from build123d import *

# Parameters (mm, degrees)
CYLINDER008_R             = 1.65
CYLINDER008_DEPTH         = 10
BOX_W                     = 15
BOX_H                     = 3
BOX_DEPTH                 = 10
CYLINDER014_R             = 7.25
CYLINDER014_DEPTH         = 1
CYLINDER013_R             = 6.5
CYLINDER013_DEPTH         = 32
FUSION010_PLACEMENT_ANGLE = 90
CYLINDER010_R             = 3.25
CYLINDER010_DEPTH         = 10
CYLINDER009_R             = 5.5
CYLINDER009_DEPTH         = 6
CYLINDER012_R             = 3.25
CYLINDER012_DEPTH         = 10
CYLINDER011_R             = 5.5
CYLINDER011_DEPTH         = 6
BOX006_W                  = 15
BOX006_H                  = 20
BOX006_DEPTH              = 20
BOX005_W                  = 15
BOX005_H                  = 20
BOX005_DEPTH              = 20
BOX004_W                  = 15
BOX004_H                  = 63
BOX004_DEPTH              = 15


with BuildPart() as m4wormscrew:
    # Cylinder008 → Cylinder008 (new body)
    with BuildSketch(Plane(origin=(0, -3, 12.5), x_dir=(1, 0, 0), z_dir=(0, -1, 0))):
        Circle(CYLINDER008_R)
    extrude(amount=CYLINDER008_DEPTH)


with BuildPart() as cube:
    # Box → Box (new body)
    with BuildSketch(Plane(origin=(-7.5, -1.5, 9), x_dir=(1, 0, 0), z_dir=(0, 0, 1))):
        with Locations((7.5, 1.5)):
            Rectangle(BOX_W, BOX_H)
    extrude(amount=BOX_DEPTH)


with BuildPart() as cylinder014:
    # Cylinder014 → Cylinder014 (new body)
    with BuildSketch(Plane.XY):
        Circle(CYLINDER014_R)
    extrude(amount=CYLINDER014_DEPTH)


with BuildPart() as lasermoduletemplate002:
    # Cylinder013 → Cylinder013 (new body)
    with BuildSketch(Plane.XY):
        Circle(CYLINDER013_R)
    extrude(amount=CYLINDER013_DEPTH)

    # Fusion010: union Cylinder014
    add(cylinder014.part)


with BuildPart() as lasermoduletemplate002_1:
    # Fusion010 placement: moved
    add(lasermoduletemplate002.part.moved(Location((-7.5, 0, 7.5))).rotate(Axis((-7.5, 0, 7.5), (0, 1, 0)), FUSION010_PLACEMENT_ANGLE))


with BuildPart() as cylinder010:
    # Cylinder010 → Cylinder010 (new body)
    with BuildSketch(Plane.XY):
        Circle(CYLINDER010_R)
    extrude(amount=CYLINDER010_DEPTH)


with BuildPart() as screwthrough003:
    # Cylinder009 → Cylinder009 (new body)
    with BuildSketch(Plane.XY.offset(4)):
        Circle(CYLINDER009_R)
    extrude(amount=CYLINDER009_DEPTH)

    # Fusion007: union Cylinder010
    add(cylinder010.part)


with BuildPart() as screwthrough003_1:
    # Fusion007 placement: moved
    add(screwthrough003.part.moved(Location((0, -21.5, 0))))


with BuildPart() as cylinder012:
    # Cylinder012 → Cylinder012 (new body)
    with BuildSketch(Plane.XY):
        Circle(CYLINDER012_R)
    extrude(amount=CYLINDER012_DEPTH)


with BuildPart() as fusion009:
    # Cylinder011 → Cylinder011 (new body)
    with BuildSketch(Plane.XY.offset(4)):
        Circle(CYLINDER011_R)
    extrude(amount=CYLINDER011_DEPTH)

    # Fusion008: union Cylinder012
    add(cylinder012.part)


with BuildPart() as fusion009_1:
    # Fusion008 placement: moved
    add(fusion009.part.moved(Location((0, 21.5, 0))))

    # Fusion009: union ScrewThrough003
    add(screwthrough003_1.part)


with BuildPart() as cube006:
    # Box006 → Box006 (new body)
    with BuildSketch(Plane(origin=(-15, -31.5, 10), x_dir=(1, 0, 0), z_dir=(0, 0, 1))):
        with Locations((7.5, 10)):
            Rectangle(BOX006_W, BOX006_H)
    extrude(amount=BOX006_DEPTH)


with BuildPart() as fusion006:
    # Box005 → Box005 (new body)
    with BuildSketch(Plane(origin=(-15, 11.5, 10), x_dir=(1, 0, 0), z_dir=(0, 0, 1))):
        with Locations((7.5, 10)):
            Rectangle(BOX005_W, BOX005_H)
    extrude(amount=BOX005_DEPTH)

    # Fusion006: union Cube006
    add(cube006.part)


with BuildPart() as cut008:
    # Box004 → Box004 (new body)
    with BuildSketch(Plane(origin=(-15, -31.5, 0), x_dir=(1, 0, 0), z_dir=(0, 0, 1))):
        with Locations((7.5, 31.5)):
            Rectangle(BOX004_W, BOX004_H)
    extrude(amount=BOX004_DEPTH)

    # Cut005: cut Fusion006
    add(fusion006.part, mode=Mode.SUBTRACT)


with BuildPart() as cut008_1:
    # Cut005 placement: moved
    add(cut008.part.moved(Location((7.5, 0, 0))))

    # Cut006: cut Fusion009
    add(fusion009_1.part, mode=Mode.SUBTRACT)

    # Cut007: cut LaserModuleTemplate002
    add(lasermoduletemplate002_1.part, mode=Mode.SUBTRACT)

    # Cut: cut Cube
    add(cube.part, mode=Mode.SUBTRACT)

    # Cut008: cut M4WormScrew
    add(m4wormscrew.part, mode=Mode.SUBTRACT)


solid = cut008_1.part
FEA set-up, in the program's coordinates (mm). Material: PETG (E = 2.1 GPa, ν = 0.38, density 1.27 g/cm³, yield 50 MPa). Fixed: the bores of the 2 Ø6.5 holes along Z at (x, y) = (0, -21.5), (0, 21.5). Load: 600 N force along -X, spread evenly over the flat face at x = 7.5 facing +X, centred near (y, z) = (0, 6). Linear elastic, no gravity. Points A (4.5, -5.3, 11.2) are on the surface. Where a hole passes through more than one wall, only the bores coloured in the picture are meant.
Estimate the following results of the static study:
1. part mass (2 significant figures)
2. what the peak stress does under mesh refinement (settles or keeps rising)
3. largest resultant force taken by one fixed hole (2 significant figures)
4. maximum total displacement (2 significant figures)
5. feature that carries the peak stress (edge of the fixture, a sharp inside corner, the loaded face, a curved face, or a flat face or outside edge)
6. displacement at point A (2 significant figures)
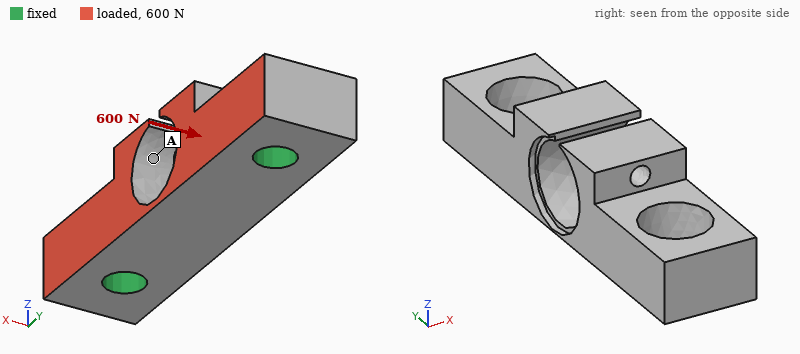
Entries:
9.7 g
keeps rising
300 N
0.18 mm
edge of the fixture
0.13 mm
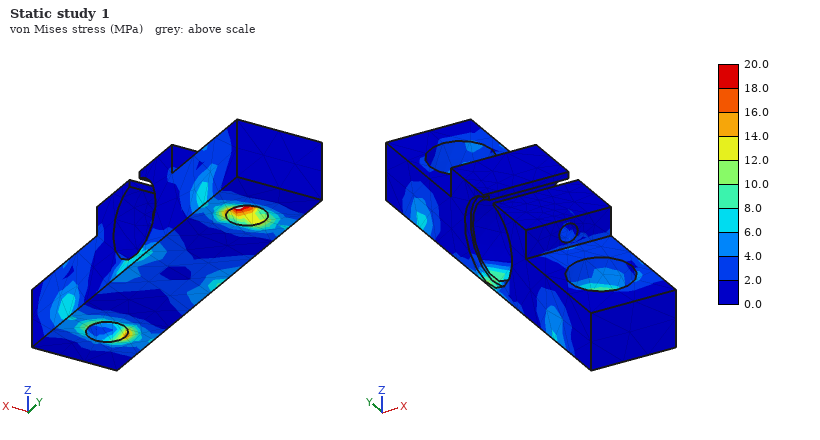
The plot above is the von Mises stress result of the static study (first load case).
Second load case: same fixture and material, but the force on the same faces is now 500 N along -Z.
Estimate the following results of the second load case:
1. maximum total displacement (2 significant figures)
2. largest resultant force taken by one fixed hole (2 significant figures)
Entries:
0.32 mm
250 N
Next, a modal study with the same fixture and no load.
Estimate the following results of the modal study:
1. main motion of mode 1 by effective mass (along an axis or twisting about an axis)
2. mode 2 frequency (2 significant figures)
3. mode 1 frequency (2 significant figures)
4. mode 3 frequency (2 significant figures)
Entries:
along Z
3600 Hz
2700 Hz
3700 Hz
